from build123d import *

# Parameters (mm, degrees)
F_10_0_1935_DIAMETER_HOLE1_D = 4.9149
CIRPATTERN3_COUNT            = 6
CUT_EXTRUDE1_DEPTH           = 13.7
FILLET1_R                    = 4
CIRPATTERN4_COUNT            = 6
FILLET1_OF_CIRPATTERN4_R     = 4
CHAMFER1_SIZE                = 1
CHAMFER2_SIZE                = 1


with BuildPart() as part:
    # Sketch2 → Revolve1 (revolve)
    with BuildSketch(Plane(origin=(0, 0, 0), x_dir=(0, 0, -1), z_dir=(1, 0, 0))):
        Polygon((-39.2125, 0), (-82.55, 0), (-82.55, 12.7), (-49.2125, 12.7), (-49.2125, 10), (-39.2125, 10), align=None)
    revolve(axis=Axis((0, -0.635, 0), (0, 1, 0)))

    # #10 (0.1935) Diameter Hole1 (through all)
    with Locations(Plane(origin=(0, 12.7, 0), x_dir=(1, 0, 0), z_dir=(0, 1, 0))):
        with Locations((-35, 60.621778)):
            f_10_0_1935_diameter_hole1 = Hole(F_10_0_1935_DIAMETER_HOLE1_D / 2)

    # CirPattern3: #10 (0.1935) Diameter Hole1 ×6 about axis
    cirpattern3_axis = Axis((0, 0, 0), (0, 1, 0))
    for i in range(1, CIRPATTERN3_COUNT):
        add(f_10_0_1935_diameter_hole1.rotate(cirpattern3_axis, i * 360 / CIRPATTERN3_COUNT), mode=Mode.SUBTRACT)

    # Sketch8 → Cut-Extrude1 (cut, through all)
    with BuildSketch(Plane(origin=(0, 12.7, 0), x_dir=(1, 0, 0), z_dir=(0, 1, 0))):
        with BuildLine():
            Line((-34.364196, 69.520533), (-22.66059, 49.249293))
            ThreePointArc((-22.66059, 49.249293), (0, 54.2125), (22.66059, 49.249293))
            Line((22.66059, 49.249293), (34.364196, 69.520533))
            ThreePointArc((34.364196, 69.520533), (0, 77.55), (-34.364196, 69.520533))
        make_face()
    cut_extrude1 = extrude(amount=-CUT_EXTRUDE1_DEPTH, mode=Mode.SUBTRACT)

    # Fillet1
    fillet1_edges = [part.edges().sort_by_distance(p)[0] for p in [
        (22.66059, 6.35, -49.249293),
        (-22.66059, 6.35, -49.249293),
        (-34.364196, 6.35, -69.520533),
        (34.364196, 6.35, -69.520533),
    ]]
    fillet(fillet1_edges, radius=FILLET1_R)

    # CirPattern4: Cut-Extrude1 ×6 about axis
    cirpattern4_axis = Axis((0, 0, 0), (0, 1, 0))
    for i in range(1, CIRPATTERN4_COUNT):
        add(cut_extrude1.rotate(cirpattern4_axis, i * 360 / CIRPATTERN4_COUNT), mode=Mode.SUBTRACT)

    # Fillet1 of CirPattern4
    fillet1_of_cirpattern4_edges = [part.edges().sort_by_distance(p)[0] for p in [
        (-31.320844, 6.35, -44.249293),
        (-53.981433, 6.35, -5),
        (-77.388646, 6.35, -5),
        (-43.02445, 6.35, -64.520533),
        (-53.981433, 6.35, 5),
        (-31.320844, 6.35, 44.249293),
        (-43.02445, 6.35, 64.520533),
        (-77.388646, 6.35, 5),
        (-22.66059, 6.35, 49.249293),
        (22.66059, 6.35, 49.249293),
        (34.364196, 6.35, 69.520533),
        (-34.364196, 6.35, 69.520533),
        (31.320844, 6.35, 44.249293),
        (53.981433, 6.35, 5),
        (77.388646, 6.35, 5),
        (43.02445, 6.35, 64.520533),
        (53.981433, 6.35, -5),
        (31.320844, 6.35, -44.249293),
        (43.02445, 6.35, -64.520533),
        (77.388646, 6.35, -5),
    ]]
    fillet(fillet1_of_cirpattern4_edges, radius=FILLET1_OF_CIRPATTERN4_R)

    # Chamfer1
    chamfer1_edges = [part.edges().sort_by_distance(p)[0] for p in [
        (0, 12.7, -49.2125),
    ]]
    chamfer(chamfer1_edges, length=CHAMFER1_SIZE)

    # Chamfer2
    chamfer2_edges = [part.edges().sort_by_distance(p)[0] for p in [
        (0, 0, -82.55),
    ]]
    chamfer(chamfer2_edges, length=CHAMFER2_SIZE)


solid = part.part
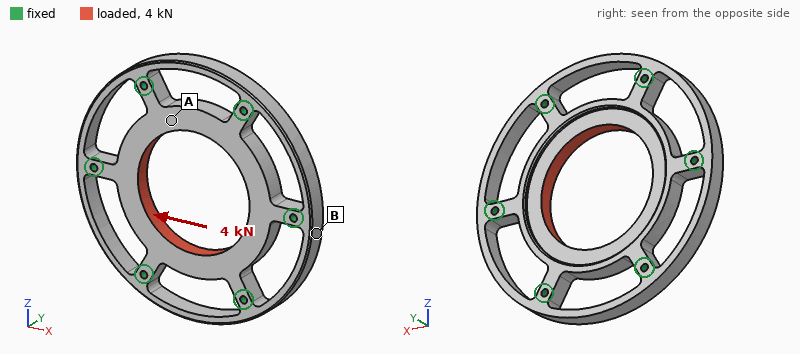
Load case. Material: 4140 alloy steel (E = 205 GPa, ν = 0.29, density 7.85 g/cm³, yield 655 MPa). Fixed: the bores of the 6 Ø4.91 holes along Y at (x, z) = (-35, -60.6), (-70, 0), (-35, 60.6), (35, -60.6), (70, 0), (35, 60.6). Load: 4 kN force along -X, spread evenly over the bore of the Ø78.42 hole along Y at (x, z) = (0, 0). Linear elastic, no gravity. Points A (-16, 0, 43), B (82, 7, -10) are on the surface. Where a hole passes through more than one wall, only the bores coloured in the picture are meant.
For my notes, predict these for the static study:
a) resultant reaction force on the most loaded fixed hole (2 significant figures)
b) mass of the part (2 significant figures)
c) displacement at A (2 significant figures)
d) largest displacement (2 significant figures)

1.1 kN
760 g
1.3 µm
1.9 µm
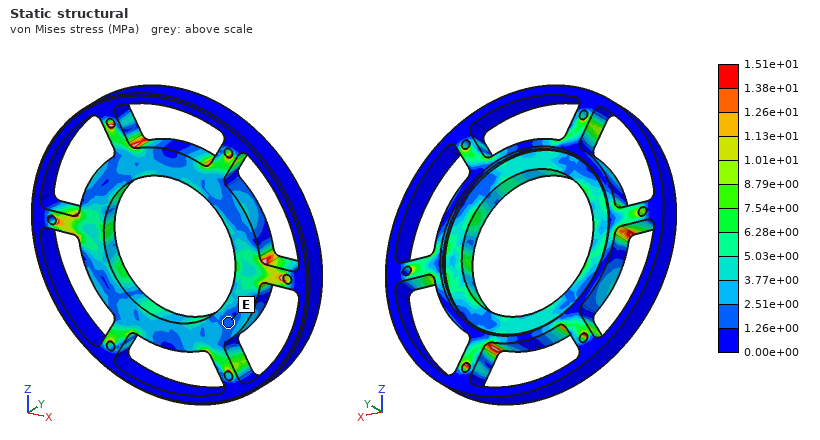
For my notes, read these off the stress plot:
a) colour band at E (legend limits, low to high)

1.26e+00 to 2.51e+00 MPa
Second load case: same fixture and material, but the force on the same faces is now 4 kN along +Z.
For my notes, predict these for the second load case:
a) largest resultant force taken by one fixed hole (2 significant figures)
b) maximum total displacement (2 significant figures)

930 N
2.1 µm
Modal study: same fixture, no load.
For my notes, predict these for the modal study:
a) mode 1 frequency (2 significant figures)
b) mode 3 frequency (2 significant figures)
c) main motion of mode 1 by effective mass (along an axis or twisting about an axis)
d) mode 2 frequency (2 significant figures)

6200 Hz
6900 Hz
along Y
6500 Hz
